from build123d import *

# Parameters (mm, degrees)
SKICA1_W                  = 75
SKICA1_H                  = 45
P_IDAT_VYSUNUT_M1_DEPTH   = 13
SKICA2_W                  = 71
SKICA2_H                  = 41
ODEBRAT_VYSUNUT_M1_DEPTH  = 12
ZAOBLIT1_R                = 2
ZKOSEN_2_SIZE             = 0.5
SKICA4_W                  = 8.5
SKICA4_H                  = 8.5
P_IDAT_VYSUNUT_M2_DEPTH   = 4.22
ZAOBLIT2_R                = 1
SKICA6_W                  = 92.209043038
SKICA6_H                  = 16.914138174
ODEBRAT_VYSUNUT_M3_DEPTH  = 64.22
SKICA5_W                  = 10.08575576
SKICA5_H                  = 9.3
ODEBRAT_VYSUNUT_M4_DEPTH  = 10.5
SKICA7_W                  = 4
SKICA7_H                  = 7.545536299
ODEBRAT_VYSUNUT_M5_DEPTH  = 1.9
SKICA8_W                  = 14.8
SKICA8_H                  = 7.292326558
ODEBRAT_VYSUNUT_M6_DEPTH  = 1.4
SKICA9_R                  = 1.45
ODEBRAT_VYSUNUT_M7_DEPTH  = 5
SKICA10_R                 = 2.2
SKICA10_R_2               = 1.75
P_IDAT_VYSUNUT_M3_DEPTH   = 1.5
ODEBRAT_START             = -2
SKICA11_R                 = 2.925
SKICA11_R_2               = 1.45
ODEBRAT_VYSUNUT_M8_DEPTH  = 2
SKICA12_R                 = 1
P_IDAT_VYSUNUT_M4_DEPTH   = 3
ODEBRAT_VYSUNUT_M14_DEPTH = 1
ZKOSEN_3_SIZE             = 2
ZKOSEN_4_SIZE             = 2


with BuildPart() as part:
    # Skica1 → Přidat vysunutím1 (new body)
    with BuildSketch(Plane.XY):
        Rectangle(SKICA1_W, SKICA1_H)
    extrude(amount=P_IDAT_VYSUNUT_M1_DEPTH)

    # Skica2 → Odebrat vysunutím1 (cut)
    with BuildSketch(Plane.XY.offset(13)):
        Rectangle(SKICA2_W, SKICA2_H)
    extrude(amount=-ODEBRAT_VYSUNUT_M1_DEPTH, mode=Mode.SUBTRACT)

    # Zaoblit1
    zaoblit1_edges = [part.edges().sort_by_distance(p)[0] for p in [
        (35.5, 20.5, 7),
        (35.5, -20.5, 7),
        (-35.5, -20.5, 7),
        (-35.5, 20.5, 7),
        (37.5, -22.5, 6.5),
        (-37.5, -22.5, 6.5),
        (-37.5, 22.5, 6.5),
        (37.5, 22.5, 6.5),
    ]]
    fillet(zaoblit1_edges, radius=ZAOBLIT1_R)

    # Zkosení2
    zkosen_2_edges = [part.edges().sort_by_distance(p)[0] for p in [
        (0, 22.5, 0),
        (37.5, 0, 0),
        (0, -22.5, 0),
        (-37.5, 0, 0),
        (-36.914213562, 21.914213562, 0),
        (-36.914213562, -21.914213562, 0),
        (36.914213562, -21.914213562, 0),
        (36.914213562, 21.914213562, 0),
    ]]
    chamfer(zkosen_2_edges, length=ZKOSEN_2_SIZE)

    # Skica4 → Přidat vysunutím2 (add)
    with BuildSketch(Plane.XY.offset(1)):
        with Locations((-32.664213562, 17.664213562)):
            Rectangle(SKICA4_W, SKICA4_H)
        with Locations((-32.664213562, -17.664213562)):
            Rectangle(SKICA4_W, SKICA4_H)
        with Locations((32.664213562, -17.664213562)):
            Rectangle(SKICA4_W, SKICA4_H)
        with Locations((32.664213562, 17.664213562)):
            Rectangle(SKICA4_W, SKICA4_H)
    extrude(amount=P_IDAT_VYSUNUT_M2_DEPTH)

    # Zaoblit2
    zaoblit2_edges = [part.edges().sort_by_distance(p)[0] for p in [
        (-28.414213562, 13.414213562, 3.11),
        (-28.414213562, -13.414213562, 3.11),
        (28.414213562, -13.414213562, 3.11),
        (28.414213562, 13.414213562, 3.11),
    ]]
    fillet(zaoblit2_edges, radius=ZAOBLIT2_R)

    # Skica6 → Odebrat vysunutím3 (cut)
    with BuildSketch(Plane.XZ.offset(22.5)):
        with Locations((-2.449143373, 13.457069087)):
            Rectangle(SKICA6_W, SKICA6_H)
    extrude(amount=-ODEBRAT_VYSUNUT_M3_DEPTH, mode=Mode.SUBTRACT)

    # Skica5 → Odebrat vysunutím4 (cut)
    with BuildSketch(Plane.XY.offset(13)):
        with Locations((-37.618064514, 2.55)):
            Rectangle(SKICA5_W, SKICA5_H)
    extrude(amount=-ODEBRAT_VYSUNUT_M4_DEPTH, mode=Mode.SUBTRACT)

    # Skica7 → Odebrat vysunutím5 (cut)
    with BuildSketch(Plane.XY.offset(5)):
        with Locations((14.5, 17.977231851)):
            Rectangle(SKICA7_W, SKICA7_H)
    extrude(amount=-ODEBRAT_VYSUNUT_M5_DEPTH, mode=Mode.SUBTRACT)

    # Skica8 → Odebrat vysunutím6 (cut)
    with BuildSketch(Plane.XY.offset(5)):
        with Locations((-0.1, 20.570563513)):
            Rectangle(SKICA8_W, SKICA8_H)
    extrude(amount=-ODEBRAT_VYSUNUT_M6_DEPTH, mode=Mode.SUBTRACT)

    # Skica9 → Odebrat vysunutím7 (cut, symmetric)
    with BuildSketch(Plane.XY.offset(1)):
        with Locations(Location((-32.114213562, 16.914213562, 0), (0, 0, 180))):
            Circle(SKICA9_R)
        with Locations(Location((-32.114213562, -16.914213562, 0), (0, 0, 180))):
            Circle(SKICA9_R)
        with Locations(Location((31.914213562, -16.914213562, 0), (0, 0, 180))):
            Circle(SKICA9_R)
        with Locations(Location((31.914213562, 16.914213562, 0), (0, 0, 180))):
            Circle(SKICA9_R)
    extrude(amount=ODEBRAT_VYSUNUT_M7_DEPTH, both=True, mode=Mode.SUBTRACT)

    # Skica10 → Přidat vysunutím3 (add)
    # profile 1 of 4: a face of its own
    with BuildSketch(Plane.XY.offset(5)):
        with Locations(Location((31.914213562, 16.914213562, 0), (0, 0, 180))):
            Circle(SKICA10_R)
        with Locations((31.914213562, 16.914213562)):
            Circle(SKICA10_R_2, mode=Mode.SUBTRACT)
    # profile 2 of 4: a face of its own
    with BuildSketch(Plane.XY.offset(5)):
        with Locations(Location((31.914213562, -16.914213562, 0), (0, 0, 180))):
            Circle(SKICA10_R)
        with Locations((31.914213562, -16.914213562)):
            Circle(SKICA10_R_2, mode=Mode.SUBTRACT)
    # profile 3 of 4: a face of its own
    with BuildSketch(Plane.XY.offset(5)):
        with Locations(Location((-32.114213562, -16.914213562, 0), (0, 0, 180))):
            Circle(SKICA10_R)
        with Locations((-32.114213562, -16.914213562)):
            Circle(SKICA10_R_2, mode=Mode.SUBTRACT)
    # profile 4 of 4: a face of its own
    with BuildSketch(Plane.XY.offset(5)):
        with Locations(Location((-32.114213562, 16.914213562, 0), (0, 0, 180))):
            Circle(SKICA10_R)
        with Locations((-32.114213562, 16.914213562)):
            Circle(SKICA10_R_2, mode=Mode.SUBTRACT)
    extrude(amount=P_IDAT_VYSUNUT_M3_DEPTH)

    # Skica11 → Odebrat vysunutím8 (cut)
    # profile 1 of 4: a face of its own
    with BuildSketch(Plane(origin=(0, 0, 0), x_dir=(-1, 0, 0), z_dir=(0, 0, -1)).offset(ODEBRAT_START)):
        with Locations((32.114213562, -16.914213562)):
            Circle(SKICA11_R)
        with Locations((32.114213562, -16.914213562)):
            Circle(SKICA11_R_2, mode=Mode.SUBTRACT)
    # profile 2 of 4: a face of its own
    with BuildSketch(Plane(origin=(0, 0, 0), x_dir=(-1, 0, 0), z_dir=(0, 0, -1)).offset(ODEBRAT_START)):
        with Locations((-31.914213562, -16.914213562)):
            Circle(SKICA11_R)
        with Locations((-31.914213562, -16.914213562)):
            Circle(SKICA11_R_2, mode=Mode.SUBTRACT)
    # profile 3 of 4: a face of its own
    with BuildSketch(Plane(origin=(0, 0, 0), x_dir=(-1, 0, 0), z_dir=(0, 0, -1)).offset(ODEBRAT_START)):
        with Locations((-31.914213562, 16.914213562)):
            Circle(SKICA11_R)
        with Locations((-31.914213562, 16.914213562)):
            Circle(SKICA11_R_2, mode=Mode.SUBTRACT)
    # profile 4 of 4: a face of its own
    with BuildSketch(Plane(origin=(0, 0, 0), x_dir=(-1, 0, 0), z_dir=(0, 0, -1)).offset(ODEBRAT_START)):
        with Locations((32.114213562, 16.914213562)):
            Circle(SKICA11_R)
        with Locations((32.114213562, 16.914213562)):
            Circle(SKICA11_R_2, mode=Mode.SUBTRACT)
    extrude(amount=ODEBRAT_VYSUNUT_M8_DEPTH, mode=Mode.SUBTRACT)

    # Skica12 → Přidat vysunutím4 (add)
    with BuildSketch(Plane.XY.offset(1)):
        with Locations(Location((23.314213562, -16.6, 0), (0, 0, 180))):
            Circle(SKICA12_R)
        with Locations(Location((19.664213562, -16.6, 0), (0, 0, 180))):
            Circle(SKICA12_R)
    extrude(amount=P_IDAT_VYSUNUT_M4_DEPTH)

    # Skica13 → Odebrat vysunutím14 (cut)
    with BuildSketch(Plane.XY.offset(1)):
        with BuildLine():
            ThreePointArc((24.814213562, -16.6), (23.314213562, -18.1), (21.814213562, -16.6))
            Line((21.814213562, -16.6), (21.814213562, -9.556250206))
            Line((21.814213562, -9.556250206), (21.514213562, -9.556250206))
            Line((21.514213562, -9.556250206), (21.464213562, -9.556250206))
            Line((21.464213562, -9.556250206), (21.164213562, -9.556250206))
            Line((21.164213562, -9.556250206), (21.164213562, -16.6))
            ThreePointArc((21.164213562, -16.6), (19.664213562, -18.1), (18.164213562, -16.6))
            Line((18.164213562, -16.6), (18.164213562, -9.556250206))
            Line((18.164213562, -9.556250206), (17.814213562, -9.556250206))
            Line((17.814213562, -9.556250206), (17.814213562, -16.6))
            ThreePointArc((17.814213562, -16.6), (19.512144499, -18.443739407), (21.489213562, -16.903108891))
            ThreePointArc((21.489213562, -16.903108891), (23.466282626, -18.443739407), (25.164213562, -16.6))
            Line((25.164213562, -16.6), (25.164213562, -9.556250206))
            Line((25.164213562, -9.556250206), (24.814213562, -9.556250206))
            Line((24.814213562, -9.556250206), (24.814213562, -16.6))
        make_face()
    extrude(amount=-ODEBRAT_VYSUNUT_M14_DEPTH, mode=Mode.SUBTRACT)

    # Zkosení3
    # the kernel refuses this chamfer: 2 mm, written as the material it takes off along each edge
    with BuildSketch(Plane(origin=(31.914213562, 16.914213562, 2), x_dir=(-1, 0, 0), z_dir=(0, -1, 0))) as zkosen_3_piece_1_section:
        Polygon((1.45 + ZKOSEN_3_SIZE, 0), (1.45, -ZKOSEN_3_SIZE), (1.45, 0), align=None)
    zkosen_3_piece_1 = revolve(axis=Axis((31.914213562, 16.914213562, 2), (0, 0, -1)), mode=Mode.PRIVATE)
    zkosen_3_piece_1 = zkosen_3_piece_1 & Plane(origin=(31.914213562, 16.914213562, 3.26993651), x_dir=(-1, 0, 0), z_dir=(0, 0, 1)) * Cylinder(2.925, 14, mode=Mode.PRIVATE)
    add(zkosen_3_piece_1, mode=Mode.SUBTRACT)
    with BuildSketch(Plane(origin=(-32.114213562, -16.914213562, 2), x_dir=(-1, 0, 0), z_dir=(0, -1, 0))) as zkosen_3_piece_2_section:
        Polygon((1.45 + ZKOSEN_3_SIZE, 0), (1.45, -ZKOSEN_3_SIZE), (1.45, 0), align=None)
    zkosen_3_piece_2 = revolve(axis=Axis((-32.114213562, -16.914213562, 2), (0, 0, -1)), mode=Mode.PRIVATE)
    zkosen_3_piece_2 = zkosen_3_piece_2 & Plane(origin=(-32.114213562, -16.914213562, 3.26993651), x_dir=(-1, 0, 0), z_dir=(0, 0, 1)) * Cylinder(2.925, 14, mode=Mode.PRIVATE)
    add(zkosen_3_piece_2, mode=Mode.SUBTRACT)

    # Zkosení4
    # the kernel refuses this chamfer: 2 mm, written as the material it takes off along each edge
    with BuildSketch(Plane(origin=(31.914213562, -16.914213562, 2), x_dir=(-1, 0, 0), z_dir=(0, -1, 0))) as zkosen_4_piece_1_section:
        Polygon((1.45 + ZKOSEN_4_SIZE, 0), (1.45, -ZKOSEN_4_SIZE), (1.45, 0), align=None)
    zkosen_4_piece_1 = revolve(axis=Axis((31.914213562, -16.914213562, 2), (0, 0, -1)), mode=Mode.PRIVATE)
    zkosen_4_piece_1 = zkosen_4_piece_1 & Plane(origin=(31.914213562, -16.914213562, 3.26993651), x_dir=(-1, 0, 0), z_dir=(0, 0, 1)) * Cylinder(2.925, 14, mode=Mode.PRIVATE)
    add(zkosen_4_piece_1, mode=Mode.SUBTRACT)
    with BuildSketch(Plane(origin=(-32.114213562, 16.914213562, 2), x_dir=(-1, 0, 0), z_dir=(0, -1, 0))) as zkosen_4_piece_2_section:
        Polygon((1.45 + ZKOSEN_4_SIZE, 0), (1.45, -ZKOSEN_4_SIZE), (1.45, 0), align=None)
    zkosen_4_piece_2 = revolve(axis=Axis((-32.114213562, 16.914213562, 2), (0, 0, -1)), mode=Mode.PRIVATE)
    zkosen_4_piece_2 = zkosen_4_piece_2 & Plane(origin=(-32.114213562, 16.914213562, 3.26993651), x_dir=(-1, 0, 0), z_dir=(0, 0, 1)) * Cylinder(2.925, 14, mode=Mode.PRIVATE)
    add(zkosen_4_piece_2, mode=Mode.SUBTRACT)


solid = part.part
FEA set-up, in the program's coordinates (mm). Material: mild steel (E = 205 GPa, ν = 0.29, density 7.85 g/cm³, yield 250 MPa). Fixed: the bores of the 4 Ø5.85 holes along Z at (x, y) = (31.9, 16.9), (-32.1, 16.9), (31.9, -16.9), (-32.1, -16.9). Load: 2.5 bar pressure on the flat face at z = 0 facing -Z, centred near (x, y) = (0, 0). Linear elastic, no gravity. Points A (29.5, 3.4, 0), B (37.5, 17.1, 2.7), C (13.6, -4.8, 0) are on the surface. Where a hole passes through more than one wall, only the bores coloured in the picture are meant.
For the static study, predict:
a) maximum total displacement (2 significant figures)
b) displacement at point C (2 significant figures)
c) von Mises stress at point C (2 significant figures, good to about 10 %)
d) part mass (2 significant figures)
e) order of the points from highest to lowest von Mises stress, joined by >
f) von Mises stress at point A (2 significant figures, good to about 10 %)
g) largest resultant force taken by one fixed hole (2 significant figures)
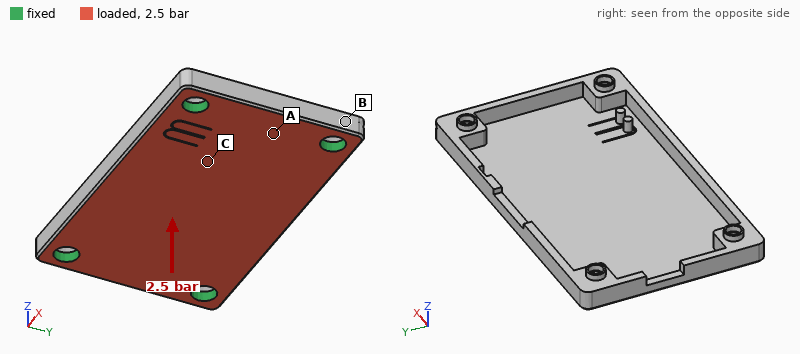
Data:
0.19 mm
0.14 mm
93 MPa
43 g
C > A > B
67 MPa
240 N
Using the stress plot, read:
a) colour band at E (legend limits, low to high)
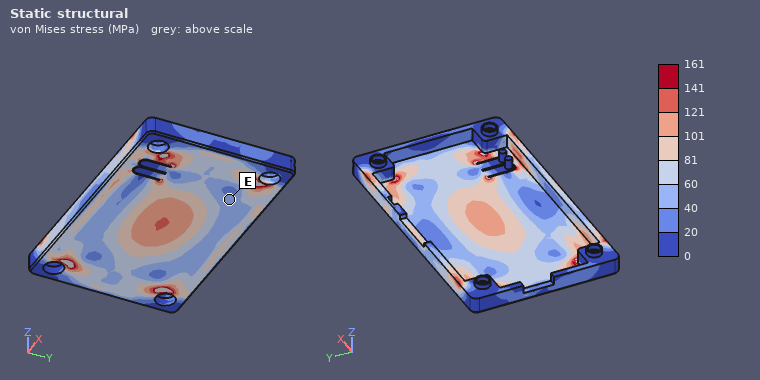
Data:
40 to 60 MPa
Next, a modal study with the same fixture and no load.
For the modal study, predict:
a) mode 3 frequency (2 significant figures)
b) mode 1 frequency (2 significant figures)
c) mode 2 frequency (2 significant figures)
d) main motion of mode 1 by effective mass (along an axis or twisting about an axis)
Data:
4900 Hz
2600 Hz
4500 Hz
along Z
